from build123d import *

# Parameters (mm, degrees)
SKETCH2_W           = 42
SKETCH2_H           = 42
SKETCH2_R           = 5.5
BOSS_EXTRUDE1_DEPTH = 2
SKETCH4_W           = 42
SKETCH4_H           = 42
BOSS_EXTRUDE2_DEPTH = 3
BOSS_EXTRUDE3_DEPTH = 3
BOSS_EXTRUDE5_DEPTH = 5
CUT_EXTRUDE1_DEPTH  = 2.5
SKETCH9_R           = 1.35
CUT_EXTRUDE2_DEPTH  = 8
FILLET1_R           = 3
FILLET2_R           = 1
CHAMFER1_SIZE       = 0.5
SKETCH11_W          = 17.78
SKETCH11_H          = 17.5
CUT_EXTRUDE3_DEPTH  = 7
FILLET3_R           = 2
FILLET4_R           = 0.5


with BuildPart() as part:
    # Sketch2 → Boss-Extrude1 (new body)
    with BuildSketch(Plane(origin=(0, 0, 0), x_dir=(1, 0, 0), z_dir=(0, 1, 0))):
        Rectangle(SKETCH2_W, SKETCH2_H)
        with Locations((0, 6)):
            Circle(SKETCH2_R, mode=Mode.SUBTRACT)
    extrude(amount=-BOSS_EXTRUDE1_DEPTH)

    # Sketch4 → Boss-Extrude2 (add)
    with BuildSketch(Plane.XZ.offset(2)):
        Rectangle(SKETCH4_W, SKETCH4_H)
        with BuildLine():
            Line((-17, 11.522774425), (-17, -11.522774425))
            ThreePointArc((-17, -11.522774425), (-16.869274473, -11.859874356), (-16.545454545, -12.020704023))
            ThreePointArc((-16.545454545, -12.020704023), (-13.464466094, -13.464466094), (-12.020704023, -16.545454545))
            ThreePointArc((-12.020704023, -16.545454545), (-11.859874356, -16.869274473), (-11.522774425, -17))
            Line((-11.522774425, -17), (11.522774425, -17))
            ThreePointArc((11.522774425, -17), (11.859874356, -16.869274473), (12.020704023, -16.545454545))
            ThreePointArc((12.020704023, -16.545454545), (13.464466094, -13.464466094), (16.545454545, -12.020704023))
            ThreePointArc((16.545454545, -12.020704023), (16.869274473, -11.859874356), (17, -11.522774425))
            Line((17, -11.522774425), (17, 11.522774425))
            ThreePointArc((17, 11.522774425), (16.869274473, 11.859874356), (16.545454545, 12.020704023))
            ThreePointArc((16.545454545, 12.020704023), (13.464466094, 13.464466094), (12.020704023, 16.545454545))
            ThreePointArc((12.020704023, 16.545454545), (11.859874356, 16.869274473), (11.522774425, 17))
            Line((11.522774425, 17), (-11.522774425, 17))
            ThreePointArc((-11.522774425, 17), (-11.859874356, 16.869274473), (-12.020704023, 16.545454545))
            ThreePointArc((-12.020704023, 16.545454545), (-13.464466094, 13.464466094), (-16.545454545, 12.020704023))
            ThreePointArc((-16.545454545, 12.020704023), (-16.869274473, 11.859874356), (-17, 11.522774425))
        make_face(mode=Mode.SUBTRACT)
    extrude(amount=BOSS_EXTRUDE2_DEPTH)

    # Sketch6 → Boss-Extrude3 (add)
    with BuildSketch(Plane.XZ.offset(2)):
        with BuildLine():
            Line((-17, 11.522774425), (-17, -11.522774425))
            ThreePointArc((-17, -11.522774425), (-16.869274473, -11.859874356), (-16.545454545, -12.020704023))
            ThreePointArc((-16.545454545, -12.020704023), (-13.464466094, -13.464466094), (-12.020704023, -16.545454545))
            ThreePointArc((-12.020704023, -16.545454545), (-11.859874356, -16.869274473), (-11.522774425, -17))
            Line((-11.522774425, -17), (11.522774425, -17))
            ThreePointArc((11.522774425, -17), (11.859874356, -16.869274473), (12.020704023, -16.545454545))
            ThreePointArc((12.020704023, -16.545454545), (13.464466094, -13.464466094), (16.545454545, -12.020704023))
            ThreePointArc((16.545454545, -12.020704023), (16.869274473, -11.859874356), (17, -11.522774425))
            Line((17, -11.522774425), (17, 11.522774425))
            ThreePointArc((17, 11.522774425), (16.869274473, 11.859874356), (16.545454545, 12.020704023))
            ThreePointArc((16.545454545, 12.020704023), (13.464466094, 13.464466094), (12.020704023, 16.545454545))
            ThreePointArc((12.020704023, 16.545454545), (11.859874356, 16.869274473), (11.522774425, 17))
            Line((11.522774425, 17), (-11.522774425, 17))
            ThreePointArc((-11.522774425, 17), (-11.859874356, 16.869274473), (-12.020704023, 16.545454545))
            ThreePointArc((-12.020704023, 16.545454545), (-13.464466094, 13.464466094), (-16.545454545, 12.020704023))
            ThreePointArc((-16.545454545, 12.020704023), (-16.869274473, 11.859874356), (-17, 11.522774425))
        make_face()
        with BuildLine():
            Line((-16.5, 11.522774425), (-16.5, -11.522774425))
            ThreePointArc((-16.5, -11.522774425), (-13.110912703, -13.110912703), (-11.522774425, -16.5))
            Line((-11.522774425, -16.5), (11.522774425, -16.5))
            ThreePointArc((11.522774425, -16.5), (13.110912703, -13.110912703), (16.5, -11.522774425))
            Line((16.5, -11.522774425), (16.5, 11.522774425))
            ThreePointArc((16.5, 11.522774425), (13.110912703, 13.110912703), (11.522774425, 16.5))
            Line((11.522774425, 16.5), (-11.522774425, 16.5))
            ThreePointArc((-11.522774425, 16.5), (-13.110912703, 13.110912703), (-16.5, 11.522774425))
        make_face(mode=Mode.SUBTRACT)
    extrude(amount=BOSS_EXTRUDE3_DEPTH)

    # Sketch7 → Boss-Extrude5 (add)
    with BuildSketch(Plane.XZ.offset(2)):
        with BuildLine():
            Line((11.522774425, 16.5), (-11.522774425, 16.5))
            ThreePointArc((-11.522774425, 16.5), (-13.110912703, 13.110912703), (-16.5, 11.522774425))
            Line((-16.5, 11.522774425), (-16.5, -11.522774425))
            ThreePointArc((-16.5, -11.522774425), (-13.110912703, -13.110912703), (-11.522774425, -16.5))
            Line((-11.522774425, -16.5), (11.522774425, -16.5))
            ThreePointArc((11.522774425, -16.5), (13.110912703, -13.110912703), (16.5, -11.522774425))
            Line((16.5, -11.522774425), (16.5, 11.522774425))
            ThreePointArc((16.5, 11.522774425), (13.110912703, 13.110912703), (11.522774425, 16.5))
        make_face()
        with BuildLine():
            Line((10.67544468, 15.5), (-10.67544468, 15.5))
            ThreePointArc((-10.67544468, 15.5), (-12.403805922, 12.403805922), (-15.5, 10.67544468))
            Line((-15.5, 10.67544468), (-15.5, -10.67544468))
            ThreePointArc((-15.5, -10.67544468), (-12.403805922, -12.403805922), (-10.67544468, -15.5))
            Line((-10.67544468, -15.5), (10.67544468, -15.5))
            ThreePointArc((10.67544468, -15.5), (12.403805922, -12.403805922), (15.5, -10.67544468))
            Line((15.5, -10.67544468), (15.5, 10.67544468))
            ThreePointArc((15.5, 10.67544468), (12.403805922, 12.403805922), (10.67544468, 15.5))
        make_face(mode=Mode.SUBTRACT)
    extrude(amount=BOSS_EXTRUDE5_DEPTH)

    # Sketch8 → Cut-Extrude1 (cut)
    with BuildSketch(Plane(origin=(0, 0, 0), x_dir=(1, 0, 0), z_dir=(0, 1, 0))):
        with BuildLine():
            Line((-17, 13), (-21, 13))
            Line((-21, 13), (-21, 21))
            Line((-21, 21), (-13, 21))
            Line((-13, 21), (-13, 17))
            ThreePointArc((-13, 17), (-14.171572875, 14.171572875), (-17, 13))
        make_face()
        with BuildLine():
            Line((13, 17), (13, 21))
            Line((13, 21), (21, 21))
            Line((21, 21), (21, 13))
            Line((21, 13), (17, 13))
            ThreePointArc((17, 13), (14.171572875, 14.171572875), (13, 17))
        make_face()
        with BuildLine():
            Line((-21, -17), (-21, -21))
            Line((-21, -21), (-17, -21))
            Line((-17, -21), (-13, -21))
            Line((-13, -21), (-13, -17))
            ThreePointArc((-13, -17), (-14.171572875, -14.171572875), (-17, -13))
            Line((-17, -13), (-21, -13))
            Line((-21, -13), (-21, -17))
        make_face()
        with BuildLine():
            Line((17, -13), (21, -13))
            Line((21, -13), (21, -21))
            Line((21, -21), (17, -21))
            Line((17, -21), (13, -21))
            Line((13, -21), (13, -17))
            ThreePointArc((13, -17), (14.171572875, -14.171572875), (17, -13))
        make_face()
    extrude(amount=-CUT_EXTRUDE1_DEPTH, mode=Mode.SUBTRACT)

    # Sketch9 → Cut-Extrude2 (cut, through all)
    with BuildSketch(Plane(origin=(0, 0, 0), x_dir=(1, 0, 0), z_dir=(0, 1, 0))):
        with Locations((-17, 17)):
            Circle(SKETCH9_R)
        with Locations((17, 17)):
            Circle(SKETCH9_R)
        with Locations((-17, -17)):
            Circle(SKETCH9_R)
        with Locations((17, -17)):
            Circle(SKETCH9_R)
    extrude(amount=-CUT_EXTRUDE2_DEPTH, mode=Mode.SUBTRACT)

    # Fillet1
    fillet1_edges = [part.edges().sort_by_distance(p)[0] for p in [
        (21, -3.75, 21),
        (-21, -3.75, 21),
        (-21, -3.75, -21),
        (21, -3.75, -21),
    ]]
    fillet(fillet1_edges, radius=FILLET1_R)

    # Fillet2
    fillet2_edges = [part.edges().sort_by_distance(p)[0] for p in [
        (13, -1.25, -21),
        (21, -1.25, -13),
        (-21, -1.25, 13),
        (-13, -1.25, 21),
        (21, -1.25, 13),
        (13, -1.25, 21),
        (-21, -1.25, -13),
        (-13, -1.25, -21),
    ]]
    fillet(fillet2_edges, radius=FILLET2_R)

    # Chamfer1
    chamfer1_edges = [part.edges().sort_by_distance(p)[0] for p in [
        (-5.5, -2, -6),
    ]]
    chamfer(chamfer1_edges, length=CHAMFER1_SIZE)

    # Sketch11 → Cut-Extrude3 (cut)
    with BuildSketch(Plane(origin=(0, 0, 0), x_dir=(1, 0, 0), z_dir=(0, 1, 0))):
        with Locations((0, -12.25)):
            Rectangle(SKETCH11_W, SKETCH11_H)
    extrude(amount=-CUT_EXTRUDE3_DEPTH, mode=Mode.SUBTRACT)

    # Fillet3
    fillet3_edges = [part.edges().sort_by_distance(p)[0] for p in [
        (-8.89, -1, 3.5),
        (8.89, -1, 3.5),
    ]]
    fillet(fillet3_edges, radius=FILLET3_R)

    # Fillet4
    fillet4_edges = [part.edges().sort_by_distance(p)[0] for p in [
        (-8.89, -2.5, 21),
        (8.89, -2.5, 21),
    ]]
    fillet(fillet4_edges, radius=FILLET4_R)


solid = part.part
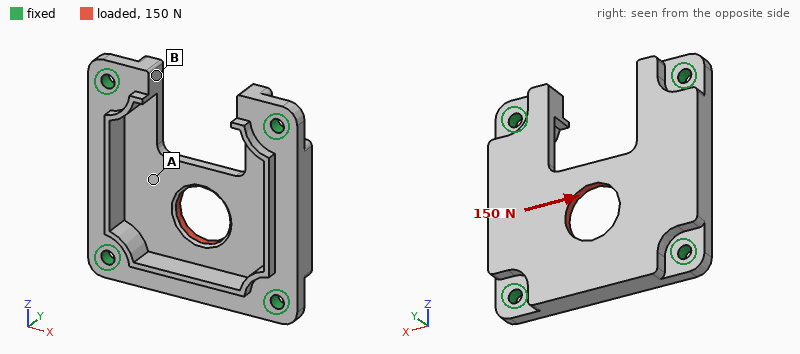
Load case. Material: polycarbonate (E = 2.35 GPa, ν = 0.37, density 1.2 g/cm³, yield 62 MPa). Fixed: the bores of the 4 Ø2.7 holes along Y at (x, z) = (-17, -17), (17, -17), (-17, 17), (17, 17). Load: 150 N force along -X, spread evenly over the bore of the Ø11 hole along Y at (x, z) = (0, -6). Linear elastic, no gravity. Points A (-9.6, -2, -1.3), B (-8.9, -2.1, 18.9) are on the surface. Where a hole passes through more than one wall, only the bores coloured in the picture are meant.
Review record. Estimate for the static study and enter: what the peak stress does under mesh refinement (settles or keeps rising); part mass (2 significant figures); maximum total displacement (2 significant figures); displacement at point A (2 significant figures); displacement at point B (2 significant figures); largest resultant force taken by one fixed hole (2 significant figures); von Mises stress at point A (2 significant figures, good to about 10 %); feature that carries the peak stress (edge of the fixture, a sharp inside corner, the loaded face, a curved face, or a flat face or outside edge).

keeps rising
5.4 g
38 µm
34 µm
15 µm
63 N
1.8 MPa
edge of the fixture
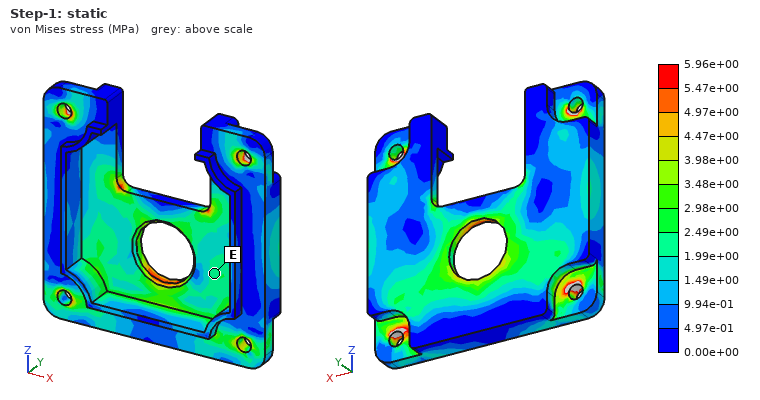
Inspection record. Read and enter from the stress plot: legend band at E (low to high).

1.99e+00 to 2.49e+00 MPa
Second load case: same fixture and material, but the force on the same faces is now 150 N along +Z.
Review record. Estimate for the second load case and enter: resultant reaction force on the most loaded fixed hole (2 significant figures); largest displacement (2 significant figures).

43 N
54 µm
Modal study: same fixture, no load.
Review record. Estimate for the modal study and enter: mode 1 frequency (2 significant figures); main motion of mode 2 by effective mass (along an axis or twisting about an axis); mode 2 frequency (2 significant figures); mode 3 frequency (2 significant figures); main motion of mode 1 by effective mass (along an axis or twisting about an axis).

3100 Hz
twisting about Z
4300 Hz
4600 Hz
along Y
